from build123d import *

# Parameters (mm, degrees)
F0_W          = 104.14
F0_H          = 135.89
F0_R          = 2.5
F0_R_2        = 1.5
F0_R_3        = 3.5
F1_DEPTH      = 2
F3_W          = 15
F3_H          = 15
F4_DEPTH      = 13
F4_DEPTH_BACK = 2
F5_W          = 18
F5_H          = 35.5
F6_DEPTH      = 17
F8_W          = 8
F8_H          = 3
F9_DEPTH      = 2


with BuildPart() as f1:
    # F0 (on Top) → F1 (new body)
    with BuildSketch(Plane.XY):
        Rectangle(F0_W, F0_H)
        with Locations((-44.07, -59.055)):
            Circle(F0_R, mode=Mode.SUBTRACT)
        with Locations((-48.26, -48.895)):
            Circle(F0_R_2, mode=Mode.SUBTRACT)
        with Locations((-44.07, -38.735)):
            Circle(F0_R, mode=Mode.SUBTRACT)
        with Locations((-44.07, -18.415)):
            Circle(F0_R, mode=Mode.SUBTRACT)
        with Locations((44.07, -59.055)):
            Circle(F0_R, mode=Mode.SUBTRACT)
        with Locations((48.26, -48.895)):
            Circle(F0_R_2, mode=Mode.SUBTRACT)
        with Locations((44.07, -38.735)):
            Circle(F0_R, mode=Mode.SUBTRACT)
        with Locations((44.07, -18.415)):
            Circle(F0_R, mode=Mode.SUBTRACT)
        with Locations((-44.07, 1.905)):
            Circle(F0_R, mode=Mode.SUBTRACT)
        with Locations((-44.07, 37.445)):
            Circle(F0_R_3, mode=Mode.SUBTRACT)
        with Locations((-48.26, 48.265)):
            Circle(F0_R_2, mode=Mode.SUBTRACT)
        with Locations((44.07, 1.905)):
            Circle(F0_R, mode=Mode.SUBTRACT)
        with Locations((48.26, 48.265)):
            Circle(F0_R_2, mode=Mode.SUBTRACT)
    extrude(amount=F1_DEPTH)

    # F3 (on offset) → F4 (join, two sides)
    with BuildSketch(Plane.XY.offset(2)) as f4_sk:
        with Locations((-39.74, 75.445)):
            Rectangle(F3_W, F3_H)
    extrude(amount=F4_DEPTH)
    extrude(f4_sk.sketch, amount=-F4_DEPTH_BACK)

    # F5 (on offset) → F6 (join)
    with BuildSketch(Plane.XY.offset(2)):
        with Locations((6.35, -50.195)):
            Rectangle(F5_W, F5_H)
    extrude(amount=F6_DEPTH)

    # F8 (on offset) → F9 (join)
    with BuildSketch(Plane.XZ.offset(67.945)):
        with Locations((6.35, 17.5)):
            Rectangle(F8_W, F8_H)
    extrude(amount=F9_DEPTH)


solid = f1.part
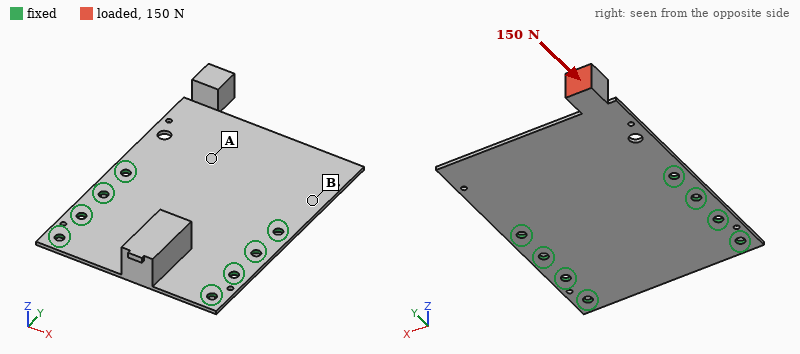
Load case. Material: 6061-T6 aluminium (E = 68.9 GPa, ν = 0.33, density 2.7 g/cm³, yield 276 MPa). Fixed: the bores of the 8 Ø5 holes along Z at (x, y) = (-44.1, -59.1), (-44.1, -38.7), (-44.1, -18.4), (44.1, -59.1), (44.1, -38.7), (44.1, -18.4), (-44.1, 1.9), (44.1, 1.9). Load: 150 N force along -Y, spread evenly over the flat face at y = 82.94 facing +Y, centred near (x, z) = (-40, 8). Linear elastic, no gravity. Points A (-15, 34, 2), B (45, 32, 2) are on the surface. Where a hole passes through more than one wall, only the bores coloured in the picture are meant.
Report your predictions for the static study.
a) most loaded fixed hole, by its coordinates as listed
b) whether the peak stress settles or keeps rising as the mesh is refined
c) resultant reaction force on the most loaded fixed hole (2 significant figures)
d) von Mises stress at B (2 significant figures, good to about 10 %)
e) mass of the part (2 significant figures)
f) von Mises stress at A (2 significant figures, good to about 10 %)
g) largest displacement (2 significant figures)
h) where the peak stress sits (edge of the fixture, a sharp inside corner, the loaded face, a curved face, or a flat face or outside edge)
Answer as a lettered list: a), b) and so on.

a) (-44.1, 1.9)
b) keeps rising
c) 100 N
d) 9.1 MPa
e) 110 g
f) 18 MPa
g) 1.2 mm
h) a sharp inside corner
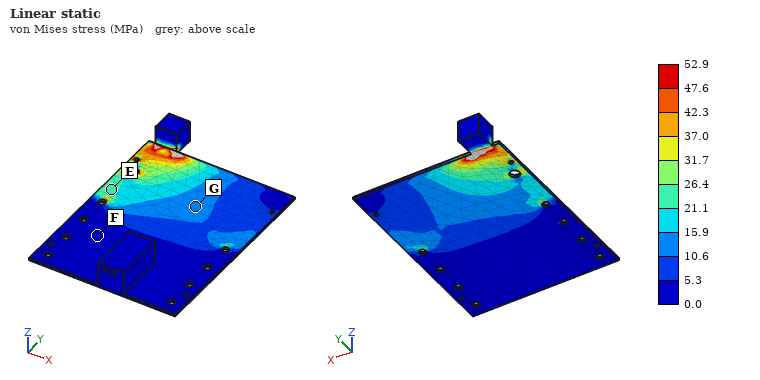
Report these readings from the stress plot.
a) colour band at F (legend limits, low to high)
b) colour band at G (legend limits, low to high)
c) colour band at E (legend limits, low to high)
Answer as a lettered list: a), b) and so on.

a) 0.0 to 5.3 MPa
b) 10.6 to 15.9 MPa
c) 21.1 to 26.4 MPa
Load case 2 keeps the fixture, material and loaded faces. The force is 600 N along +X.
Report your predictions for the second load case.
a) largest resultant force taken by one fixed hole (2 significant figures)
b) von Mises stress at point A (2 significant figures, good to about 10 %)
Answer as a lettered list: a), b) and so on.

a) 520 N
b) 56 MPa
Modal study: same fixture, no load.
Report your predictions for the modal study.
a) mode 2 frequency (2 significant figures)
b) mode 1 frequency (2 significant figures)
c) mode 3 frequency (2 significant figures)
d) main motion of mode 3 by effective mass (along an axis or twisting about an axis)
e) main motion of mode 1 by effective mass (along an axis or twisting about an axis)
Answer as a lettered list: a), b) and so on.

a) 500 Hz
b) 200 Hz
c) 890 Hz
d) along Z
e) along Z
